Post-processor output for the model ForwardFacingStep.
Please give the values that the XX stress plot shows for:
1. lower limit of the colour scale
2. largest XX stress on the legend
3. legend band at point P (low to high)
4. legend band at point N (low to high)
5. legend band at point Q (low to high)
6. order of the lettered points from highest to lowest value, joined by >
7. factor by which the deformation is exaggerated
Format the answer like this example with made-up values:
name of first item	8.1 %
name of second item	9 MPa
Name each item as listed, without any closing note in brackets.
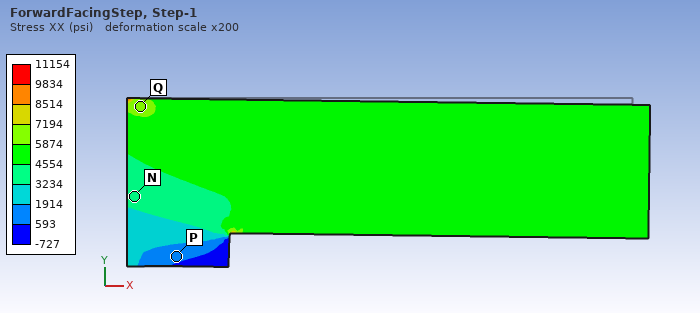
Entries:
lower limit of the colour scale	-727 psi
largest XX stress on the legend	11154 psi
legend band at point P	593 to 1914 psi
legend band at point N	3234 to 4554 psi
legend band at point Q	5874 to 7194 psi
order of the lettered points from highest to lowest value, joined by >	Q > N > P
factor by which the deformation is exaggerated	200
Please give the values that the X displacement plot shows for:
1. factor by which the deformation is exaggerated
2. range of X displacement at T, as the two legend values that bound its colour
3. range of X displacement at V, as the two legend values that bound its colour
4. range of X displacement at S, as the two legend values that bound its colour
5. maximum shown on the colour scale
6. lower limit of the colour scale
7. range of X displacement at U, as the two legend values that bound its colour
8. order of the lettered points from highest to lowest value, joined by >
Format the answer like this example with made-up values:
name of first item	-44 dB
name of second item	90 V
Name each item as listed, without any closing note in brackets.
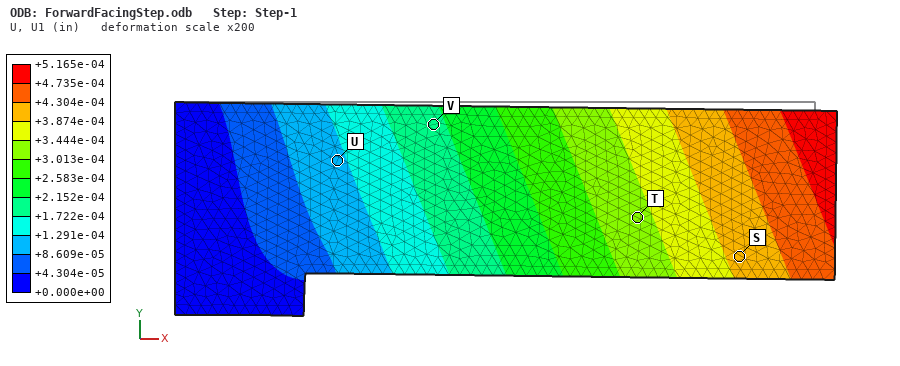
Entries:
factor by which the deformation is exaggerated	200
range of X displacement at T, as the two legend values that bound its colour	+3.013e-04 to +3.444e-04 in
range of X displacement at V, as the two legend values that bound its colour	+1.722e-04 to +2.152e-04 in
range of X displacement at S, as the two legend values that bound its colour	+3.874e-04 to +4.304e-04 in
maximum shown on the colour scale	+5.165e-04 in
lower limit of the colour scale	+0.000e+00 in
range of X displacement at U, as the two legend values that bound its colour	+8.609e-05 to +1.291e-04 in
order of the lettered points from highest to lowest value, joined by >	S > T > V > U
